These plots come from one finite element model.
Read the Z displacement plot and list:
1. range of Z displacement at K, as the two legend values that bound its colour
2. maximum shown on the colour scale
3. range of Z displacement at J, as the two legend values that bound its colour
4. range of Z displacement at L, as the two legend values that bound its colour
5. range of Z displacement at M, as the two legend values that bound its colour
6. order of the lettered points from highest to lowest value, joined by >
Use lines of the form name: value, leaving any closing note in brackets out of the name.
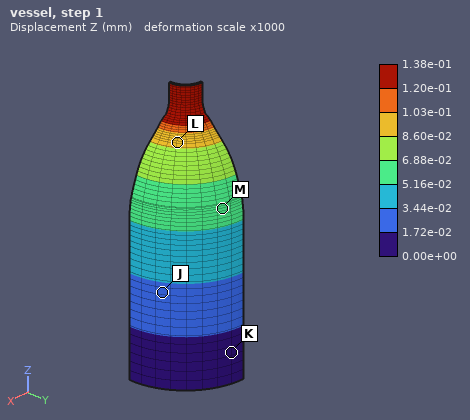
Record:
range of Z displacement at K, as the two legend values that bound its colour: 0.00e+00 to 1.72e-02 mm
maximum shown on the colour scale: 1.38e-01 mm
range of Z displacement at J, as the two legend values that bound its colour: 1.72e-02 to 3.44e-02 mm
range of Z displacement at L, as the two legend values that bound its colour: 8.60e-02 to 1.03e-01 mm
range of Z displacement at M, as the two legend values that bound its colour: 5.16e-02 to 6.88e-02 mm
order of the lettered points from highest to lowest value, joined by >: L > M > J > K
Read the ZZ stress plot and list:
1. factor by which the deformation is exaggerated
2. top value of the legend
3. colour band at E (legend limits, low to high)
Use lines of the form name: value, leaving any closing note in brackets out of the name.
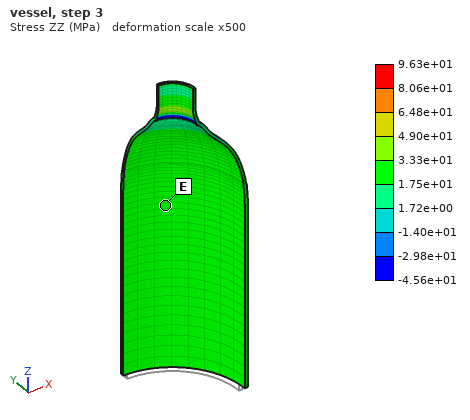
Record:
factor by which the deformation is exaggerated: 500
top value of the legend: 9.63e+01 MPa
colour band at E: 1.75e+01 to 3.33e+01 MPa
